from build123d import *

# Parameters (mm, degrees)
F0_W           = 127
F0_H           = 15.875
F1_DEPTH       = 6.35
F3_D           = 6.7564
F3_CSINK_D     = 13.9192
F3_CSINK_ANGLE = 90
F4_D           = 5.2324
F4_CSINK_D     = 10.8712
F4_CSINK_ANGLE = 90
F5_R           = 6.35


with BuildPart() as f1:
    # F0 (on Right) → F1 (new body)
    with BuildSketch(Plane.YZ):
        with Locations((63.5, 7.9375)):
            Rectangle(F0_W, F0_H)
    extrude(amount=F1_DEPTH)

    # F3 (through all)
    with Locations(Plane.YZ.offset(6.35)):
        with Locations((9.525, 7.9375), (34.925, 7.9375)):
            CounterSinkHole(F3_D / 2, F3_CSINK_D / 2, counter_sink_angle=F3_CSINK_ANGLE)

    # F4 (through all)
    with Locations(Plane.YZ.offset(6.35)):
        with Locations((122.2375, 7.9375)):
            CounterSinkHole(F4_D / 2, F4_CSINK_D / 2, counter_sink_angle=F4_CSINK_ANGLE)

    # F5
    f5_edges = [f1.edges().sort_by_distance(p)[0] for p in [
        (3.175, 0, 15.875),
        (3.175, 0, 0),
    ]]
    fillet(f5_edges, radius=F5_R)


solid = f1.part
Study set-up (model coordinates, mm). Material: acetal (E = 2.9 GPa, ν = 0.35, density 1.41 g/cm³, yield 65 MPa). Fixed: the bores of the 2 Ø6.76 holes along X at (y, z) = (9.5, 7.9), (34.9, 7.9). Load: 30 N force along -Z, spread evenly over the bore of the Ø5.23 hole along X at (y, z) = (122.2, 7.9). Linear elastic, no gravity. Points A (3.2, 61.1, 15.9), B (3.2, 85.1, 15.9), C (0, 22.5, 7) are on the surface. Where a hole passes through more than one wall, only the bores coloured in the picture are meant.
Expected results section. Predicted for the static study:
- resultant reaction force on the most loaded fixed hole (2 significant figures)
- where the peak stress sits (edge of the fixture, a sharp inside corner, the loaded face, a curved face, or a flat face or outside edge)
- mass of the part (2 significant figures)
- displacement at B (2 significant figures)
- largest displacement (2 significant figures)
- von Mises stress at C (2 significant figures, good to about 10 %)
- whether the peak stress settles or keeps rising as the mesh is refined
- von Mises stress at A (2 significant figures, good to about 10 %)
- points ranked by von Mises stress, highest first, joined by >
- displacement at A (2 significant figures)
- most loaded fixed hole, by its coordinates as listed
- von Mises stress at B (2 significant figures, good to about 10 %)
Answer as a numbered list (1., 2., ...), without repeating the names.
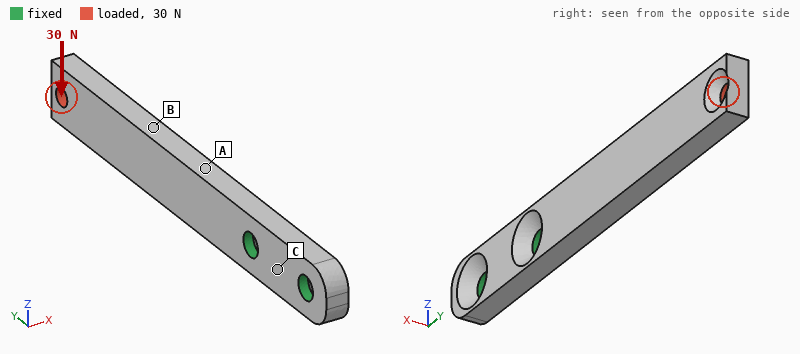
1. 77 N
2. edge of the fixture
3. 16 g
4. 0.59 mm
5. 1.5 mm
6. 1.5 MPa
7. keeps rising
8. 6.9 MPa
9. A > B > C
10. 0.22 mm
11. (34.9, 7.9)
12. 4.2 MPa
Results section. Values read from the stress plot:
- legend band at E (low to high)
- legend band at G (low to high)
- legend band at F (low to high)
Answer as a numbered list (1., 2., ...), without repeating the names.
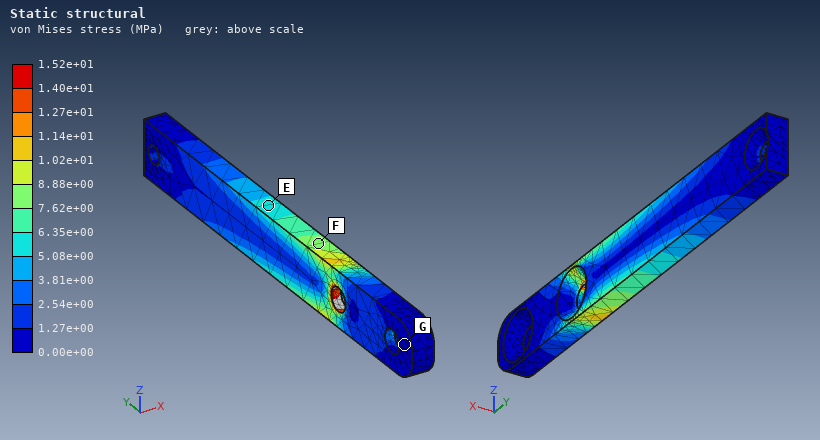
1. 5.08e+00 to 6.35e+00 MPa
2. 0.00e+00 to 1.27e+00 MPa
3. 7.62e+00 to 8.88e+00 MPa
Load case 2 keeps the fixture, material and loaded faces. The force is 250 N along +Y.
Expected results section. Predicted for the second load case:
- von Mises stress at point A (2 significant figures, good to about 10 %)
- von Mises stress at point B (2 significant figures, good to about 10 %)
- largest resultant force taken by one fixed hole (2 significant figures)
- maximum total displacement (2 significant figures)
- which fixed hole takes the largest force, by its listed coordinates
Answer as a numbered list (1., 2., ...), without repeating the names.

1. 2.5 MPa
2. 2.5 MPa
3. 230 N
4. 1.4 mm
5. (34.9, 7.9)
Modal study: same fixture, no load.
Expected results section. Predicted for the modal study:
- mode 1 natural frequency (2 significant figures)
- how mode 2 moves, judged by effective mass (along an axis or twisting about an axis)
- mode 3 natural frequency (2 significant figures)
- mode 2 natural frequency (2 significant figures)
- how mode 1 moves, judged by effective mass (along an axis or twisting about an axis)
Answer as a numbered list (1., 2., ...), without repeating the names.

1. 160 Hz
2. along Z
3. 1000 Hz
4. 400 Hz
5. along X
